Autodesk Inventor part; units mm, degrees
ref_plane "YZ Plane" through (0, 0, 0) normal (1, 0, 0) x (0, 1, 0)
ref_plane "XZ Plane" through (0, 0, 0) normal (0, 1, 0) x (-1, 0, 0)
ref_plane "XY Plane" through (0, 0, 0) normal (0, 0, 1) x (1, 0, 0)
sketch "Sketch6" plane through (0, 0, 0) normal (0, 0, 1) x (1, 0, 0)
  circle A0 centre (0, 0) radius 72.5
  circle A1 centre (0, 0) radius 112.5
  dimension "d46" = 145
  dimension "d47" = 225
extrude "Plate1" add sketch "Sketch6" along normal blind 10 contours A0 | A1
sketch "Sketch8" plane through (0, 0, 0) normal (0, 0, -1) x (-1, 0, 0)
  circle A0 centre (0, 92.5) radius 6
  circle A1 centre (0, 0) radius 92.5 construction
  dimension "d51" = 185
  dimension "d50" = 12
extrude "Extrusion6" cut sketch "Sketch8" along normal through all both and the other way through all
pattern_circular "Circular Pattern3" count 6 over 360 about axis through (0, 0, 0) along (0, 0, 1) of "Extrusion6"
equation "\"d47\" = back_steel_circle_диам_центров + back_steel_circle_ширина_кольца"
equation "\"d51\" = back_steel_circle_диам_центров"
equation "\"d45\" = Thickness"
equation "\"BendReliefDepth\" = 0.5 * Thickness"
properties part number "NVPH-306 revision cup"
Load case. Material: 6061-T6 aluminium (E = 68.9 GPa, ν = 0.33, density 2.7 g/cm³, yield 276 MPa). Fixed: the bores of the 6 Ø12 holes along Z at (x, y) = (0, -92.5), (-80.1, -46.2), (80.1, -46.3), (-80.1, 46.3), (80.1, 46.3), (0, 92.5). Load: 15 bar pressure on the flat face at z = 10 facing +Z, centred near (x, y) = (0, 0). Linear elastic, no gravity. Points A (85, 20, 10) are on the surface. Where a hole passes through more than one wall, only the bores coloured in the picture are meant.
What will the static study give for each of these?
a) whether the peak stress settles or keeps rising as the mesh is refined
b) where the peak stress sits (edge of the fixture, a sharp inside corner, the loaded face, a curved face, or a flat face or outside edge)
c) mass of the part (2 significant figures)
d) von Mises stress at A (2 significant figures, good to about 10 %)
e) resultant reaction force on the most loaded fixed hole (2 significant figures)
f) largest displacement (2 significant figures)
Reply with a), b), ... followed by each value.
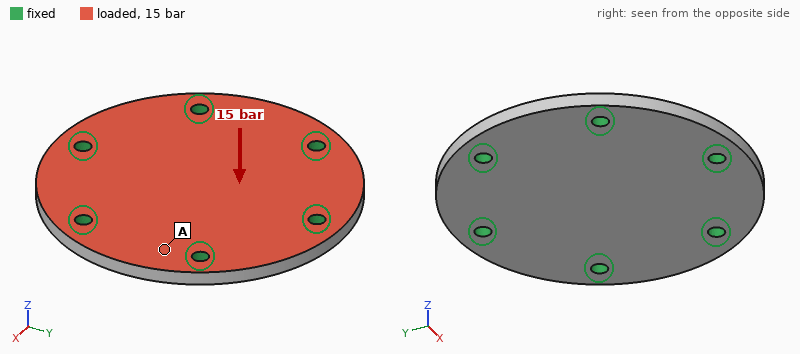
a) keeps rising
b) edge of the fixture
c) 1.1 kg
d) 41 MPa
e) 9.8 kN
f) 0.33 mm
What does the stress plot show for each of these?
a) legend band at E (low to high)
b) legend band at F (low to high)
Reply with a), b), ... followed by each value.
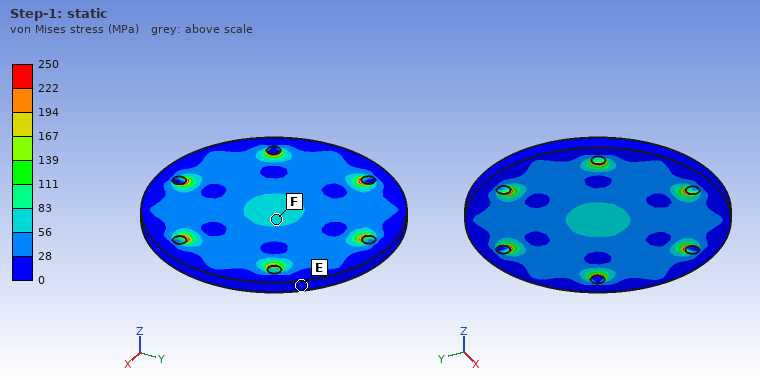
a) 0 to 28 MPa
b) 56 to 83 MPa
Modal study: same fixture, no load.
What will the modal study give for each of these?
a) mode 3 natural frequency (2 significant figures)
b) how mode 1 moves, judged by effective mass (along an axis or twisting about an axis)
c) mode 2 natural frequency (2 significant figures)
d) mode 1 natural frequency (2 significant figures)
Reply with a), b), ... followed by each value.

a) 5000 Hz
b) along Z
c) 5000 Hz
d) 2500 Hz
